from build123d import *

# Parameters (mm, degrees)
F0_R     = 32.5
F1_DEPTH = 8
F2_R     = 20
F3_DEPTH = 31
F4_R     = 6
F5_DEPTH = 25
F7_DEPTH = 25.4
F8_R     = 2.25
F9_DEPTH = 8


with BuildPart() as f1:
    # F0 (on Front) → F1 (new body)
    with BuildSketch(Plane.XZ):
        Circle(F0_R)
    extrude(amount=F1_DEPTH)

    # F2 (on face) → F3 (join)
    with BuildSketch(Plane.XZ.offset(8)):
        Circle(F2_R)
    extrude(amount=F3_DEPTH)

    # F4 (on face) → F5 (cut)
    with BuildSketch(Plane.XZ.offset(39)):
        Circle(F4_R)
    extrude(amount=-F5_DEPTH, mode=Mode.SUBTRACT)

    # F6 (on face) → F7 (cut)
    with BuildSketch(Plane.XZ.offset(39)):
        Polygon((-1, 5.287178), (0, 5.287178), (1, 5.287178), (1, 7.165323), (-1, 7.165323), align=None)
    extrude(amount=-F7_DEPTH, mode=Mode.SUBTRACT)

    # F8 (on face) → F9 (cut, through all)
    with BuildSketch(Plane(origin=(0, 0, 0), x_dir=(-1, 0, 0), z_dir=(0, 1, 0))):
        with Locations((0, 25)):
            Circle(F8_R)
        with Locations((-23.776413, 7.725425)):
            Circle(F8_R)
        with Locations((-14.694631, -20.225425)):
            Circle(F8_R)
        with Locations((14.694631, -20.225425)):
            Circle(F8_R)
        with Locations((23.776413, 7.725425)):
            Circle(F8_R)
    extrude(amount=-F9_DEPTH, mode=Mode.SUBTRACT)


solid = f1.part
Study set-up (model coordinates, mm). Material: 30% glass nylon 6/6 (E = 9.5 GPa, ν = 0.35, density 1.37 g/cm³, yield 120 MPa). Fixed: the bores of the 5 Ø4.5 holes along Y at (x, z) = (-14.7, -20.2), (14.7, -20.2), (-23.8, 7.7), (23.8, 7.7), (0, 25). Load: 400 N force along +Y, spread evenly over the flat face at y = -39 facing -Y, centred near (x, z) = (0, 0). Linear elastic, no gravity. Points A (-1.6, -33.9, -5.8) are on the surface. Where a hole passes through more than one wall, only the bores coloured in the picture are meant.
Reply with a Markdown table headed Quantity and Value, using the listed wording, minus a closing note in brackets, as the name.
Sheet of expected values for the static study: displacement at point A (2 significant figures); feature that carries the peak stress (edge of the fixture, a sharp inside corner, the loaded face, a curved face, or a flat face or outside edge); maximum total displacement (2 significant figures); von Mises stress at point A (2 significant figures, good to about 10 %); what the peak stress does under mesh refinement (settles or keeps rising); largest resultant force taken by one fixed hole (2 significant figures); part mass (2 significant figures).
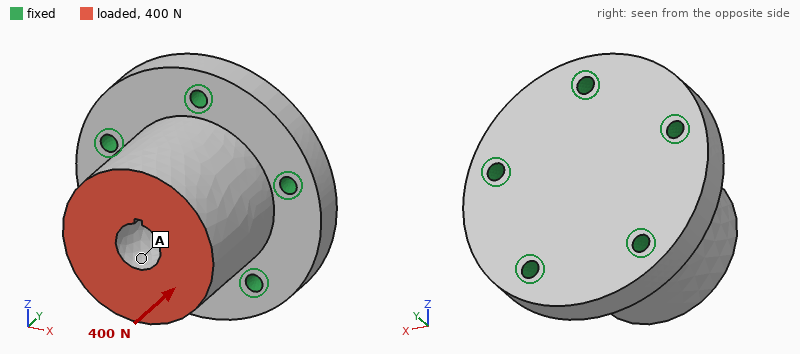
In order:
| Quantity | Value |
|---|---|
| displacement at point A | 2.8 µm |
| feature that carries the peak stress | edge of the fixture |
| maximum total displacement | 3.1 µm |
| von Mises stress at point A | 0.35 MPa |
| what the peak stress does under mesh refinement | keeps rising |
| largest resultant force taken by one fixed hole | 85 N |
| part mass | 85 g |
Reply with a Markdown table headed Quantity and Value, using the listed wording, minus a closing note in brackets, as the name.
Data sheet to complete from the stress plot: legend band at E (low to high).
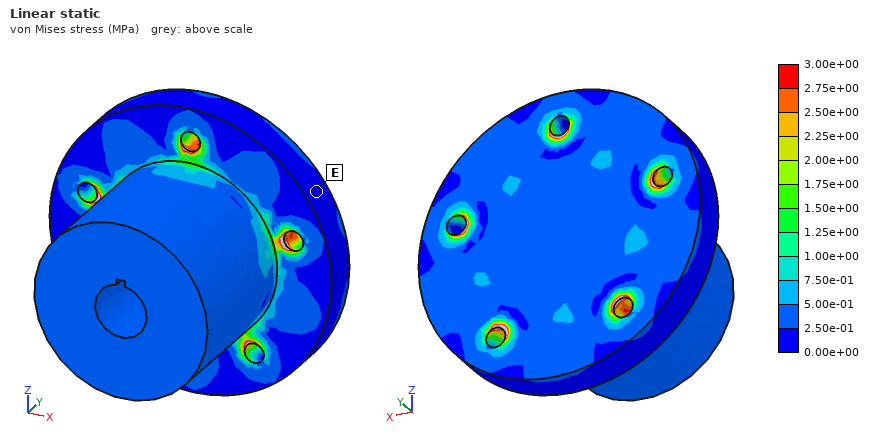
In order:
| Quantity | Value |
|---|---|
| legend band at E | 0.00e+00 to 2.50e-01 MPa |
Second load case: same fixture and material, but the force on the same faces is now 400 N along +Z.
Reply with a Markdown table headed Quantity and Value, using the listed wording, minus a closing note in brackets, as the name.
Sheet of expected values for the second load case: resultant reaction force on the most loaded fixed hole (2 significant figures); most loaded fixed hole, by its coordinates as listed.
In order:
| Quantity | Value |
|---|---|
| resultant reaction force on the most loaded fixed hole | 260 N |
| most loaded fixed hole, by its coordinates as listed | (0, 25) |
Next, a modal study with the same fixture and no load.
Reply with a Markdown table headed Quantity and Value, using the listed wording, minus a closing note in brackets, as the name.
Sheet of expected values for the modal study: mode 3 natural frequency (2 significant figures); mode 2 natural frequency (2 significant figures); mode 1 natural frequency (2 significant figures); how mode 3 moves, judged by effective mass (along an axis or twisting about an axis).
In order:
| Quantity | Value |
|---|---|
| mode 3 natural frequency | 8300 Hz |
| mode 2 natural frequency | 5600 Hz |
| mode 1 natural frequency | 5600 Hz |
| how mode 3 moves, judged by effective mass | along Y |
